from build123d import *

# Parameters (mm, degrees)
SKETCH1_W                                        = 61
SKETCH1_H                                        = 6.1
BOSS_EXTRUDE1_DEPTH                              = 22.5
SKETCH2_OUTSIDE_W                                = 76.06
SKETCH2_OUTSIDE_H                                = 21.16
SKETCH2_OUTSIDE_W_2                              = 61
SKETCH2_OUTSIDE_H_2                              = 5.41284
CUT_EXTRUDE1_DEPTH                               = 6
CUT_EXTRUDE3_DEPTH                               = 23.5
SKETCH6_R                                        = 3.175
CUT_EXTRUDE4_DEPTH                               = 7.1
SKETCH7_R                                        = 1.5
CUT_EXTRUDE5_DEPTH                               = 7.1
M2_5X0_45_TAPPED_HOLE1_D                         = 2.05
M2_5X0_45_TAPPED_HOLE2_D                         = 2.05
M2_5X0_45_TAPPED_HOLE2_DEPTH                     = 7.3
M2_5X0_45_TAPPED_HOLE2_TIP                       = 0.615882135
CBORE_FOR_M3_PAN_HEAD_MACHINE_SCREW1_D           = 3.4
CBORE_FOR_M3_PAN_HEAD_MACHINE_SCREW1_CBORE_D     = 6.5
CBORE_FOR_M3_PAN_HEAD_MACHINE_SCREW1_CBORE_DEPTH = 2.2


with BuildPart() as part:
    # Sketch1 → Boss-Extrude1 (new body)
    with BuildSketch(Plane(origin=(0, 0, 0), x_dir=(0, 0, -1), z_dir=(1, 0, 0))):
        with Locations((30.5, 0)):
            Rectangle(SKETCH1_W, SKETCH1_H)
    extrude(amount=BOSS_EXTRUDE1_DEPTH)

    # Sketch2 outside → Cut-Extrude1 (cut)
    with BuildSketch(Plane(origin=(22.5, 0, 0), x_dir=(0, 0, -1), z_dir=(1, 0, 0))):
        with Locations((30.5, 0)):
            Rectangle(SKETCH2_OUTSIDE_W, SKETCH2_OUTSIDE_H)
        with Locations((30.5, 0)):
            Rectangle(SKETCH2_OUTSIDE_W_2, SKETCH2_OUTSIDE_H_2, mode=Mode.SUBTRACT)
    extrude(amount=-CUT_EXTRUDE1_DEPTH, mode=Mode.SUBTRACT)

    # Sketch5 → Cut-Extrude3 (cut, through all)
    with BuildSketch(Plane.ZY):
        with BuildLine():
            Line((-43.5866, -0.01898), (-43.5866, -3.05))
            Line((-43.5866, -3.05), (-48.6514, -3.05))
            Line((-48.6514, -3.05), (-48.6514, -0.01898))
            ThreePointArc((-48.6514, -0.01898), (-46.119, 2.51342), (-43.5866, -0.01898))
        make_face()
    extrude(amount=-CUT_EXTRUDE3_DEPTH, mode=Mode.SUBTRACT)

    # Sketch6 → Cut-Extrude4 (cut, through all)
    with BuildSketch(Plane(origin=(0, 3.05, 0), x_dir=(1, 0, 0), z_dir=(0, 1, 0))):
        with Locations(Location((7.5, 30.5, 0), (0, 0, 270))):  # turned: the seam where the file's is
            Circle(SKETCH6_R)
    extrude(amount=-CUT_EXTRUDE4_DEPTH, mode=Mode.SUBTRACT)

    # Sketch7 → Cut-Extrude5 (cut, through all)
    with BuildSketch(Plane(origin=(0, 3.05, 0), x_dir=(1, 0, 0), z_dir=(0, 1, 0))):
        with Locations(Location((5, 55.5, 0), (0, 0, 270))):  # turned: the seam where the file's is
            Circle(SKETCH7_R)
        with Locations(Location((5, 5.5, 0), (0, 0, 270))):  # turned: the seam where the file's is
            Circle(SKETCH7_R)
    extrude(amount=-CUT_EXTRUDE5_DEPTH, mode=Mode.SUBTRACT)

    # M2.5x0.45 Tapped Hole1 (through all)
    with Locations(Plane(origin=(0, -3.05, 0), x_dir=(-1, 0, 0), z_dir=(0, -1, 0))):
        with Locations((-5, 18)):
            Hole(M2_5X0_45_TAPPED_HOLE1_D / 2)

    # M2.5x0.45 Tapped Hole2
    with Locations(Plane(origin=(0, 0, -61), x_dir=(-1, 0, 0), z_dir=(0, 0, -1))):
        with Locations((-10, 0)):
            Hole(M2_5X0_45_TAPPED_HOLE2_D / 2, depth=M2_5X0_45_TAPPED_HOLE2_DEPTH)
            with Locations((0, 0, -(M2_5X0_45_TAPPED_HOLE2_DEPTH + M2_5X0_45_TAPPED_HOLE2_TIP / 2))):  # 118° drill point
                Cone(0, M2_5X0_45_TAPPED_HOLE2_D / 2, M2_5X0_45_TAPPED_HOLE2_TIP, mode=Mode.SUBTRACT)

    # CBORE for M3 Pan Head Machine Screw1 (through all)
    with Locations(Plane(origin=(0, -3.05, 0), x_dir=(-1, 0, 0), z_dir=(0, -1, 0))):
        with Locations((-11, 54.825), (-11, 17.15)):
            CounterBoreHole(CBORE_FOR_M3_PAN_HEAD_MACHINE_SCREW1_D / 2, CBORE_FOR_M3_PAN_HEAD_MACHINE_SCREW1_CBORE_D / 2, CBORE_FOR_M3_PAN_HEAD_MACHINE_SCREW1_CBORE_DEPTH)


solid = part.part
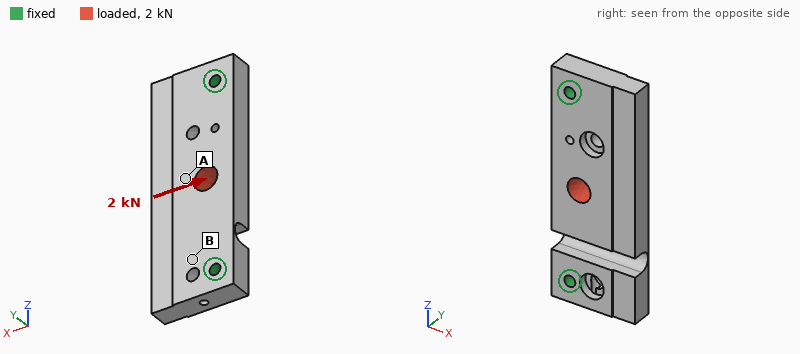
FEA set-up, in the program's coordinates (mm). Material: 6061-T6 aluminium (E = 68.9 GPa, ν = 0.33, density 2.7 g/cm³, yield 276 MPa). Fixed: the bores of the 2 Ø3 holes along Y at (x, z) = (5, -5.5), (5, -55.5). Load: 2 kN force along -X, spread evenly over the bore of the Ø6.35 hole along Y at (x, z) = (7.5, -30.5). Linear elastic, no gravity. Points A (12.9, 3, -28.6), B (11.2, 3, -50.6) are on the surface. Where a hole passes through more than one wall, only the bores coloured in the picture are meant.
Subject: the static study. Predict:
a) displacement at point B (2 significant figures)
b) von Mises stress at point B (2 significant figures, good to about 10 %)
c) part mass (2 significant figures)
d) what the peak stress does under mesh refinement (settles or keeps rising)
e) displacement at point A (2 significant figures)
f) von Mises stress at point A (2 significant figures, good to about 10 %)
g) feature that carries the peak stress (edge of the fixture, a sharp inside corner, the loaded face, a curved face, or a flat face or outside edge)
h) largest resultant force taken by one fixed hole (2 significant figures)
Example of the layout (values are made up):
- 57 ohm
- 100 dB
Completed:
- 11 µm
- 49 MPa
- 19 g
- keeps rising
- 27 µm
- 26 MPa
- a sharp inside corner
- 1.1 kN
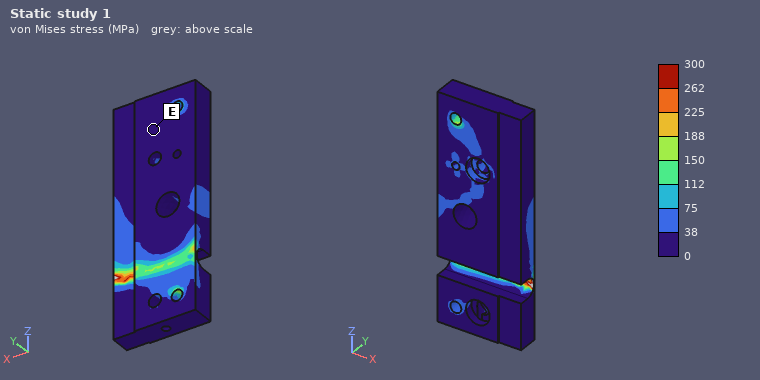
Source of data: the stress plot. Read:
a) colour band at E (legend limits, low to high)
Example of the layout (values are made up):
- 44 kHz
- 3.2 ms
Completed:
- 0 to 38 MPa
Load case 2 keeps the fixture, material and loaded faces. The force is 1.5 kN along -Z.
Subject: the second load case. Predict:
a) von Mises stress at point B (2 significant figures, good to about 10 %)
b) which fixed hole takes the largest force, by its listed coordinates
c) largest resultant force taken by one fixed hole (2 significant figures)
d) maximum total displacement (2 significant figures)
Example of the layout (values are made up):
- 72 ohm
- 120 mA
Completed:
- 12 MPa
- (5, -5.5)
- 1.2 kN
- 10 µm
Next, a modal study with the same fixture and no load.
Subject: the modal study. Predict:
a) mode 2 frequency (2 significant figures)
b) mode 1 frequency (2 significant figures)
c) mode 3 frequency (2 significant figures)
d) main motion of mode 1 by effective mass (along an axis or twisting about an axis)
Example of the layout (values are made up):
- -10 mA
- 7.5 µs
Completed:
- 9300 Hz
- 6200 Hz
- 12 kHz
- along Y
